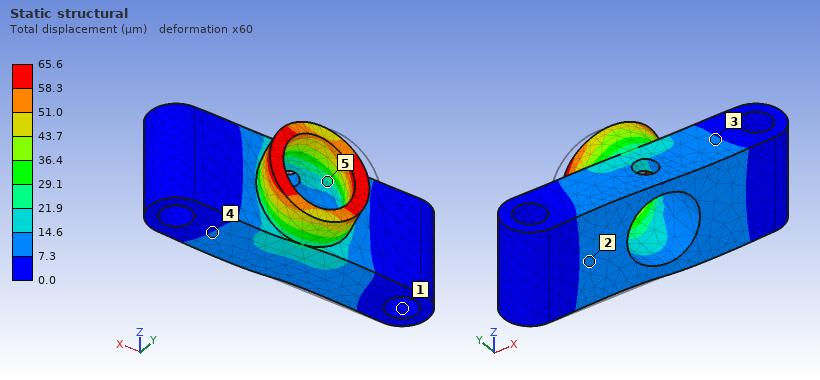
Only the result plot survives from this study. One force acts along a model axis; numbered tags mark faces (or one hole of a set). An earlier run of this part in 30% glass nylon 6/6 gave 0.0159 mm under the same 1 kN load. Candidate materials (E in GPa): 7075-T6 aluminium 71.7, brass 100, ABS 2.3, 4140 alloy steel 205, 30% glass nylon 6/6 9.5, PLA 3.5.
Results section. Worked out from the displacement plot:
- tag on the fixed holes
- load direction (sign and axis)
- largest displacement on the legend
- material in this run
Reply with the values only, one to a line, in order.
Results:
1
+X
65.6 µm
ABS
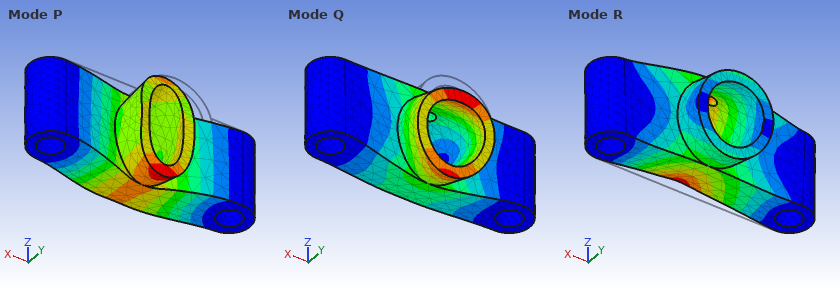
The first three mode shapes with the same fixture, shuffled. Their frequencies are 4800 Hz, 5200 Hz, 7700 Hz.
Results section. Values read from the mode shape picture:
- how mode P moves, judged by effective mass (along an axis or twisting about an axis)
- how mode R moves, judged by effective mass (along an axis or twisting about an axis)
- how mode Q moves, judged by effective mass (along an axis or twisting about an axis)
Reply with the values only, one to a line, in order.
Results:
along Y
along Z
along Z
